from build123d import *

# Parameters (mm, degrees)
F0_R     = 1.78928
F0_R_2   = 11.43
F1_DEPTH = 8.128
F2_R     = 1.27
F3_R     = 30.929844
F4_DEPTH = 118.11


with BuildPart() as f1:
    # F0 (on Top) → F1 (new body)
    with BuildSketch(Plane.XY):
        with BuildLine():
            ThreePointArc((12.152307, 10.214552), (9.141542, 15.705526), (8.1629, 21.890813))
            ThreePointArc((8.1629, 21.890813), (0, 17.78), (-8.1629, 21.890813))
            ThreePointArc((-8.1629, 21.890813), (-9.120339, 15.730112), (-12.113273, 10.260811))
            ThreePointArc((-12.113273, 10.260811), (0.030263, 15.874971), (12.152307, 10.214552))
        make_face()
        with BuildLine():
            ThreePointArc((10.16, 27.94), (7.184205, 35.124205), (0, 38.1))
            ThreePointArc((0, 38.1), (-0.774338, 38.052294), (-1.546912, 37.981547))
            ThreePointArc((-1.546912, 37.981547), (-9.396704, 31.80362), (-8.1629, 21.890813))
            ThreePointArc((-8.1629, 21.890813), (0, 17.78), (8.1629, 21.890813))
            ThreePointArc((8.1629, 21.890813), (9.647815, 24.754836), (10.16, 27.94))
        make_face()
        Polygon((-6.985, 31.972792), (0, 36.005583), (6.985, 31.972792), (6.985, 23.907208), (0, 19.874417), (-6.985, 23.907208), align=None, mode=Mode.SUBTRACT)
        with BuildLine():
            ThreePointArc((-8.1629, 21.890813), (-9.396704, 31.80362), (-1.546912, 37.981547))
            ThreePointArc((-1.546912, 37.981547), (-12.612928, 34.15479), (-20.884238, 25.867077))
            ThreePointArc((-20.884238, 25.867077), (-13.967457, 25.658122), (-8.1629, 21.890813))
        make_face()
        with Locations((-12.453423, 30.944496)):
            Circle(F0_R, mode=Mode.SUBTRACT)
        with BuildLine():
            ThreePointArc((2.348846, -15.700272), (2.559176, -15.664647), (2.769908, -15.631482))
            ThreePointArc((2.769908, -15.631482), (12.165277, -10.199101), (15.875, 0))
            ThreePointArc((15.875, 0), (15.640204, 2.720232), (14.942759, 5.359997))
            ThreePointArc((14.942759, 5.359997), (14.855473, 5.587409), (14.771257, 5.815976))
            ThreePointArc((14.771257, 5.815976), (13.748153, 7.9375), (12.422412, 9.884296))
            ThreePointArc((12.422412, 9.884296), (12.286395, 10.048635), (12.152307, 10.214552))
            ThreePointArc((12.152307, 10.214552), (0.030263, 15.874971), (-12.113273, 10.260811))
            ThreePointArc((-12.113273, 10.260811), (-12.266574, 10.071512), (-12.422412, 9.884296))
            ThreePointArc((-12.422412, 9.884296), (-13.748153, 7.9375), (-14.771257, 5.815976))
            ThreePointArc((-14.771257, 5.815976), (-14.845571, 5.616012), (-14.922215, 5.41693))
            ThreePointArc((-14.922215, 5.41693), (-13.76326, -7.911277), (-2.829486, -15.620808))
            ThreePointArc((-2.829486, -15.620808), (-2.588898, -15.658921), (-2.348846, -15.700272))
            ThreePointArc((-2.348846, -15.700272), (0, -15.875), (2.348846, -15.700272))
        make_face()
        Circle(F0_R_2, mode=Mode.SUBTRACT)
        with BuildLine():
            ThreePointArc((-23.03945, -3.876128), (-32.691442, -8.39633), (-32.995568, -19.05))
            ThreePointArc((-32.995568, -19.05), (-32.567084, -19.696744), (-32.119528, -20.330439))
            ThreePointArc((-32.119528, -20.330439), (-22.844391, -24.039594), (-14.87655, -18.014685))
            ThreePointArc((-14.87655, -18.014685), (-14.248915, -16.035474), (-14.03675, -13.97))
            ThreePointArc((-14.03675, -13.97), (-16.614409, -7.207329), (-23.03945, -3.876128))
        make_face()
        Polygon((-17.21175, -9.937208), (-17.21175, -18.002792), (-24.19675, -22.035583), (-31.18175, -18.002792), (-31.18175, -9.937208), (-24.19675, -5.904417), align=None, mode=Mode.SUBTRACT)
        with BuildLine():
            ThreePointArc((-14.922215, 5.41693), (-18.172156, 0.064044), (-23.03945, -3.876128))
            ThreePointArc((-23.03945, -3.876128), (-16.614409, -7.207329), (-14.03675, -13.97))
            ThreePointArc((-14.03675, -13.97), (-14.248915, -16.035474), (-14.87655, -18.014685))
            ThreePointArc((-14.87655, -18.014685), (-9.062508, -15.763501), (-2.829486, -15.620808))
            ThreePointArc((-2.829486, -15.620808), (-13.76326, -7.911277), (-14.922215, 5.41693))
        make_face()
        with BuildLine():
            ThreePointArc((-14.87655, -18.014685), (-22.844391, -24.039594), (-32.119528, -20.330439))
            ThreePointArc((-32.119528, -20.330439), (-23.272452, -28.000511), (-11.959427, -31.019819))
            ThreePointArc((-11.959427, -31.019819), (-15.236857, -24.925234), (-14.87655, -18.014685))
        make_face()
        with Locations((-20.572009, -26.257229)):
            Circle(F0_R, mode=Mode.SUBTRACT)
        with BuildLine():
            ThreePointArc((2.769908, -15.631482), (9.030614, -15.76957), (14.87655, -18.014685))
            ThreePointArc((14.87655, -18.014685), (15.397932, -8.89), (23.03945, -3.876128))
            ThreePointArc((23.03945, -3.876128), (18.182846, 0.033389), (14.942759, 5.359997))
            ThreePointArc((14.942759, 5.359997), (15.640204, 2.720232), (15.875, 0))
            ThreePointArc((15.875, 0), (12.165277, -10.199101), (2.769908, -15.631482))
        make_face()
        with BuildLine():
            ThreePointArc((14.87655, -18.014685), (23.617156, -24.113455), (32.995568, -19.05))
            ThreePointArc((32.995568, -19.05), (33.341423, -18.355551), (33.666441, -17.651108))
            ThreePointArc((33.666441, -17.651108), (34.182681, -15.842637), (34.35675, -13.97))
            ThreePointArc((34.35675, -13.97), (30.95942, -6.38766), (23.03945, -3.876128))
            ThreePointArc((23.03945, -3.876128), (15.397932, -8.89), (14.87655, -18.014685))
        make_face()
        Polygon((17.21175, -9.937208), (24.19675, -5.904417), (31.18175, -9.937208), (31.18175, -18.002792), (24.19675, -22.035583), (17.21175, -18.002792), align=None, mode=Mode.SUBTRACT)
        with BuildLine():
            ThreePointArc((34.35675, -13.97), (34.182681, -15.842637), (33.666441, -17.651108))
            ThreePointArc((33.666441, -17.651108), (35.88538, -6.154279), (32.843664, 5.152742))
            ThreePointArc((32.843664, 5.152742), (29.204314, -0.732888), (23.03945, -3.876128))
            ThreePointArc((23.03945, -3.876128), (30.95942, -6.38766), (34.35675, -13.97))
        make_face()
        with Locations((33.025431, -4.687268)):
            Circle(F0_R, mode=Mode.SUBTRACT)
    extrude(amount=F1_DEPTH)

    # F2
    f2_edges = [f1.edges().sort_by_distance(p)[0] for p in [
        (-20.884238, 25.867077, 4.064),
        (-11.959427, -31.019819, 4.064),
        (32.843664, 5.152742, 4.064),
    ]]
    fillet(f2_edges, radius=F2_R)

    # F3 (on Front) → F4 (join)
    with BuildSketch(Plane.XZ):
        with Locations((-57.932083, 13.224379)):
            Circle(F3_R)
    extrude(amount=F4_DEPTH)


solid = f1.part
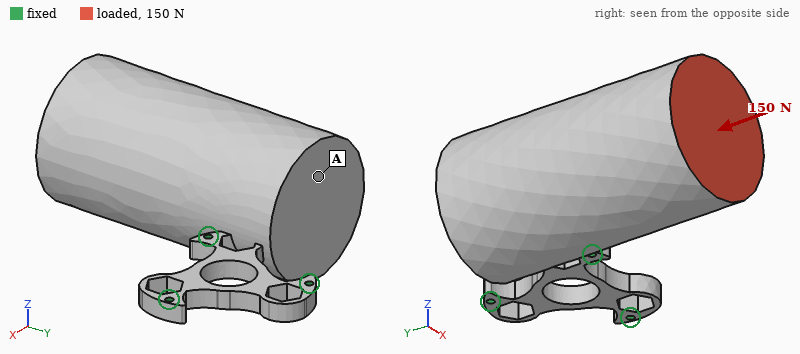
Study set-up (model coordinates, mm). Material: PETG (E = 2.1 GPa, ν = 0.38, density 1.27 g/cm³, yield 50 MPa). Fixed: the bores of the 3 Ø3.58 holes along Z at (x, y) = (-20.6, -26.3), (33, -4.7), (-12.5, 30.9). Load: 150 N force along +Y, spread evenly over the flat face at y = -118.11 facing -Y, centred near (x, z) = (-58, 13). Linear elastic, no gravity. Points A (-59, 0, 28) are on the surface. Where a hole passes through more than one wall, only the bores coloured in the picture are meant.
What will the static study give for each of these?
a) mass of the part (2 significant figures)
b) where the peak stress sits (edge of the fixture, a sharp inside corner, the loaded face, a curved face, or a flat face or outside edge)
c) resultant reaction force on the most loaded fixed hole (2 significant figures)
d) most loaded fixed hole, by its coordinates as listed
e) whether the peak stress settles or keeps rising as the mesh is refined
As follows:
460 g
edge of the fixture
240 N
(-20.6, -26.3)
keeps rising
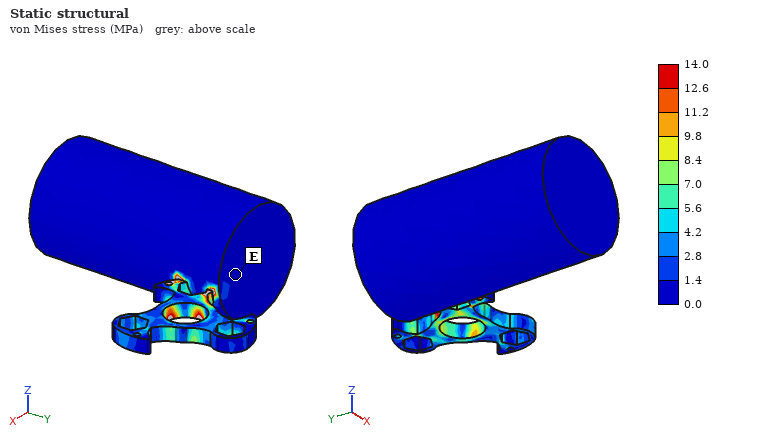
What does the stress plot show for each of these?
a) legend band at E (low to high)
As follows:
0.0 to 1.4 MPa
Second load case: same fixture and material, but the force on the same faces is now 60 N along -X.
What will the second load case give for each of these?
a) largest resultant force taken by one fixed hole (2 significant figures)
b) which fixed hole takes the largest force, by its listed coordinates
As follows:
270 N
(-20.6, -26.3)
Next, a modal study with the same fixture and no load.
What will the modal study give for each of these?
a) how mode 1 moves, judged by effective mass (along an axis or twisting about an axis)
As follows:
along Z
